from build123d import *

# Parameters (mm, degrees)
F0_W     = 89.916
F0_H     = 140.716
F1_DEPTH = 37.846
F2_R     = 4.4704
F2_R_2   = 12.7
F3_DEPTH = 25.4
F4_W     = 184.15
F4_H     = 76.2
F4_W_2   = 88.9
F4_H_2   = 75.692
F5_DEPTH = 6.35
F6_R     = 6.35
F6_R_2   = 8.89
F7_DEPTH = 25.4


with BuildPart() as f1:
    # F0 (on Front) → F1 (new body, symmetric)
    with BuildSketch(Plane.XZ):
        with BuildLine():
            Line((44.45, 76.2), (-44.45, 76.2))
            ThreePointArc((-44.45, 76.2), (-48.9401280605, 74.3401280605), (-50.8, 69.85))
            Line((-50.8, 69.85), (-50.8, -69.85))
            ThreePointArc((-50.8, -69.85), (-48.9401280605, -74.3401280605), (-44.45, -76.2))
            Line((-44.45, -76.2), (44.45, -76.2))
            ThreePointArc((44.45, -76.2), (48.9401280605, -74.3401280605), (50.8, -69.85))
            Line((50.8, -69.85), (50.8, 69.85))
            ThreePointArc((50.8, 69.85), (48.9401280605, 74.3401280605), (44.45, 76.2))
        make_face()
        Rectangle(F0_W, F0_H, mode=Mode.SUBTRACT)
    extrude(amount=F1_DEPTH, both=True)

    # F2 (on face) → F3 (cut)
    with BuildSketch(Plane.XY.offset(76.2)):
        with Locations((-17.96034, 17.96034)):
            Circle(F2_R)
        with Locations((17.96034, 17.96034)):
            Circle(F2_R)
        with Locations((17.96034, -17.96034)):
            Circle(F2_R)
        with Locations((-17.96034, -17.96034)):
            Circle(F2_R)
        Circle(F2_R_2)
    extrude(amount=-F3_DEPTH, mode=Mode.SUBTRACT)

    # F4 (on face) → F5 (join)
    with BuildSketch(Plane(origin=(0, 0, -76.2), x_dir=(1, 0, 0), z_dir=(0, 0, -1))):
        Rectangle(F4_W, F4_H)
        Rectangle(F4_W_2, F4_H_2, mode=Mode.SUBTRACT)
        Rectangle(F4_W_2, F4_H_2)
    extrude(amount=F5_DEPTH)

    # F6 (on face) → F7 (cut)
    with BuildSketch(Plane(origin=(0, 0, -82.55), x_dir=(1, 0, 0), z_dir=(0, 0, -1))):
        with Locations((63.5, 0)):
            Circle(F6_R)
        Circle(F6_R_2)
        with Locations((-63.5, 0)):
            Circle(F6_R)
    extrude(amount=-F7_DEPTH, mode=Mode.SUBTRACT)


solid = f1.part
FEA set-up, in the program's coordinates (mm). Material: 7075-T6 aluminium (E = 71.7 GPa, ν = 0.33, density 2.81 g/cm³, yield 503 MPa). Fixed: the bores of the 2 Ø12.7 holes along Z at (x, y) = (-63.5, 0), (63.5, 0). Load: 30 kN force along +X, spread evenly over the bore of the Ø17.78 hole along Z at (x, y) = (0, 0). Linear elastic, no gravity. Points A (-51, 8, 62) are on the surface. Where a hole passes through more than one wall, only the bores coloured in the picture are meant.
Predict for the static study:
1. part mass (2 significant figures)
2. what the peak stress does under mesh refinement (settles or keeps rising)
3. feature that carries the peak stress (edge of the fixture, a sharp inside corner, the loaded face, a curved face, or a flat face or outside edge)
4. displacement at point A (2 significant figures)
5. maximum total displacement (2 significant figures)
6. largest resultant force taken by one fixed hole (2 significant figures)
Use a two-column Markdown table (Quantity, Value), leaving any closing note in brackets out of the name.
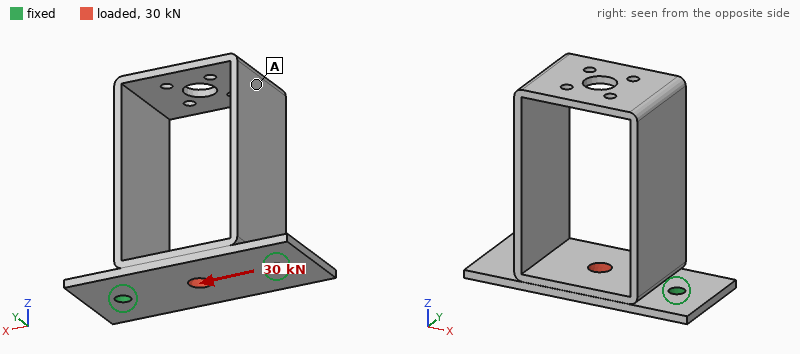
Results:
| Quantity | Value |
|---|---|
| part mass | 820 g |
| what the peak stress does under mesh refinement | keeps rising |
| feature that carries the peak stress | edge of the fixture |
| displacement at point A | 82 µm |
| maximum total displacement | 84 µm |
| largest resultant force taken by one fixed hole | 15 kN |
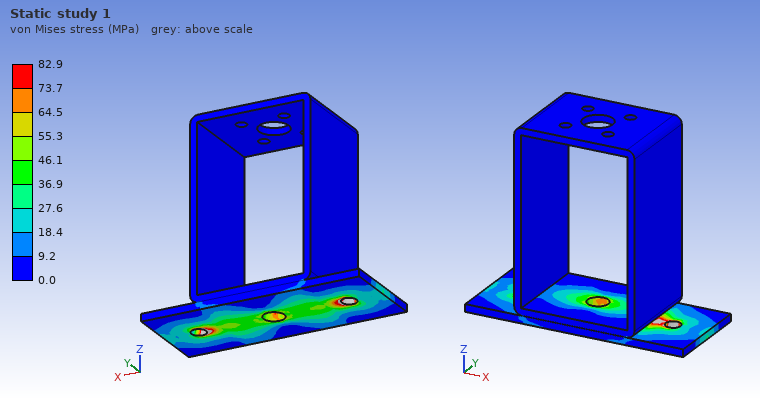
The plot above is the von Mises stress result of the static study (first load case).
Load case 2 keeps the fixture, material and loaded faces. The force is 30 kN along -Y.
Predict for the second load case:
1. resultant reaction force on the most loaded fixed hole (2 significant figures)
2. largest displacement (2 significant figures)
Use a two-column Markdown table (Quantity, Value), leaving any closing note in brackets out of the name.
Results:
| Quantity | Value |
|---|---|
| resultant reaction force on the most loaded fixed hole | 15 kN |
| largest displacement | 0.58 mm |
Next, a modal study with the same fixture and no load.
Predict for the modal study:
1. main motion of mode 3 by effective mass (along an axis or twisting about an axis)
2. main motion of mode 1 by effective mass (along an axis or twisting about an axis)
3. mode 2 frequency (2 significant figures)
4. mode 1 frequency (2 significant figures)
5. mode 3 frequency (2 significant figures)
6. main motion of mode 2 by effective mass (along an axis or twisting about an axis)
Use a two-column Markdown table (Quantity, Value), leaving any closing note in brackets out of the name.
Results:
| Quantity | Value |
|---|---|
| main motion of mode 3 by effective mass | twisting about Z |
| main motion of mode 1 by effective mass | along X |
| mode 2 frequency | 340 Hz |
| mode 1 frequency | 230 Hz |
| mode 3 frequency | 740 Hz |
| main motion of mode 2 by effective mass | along Y |
